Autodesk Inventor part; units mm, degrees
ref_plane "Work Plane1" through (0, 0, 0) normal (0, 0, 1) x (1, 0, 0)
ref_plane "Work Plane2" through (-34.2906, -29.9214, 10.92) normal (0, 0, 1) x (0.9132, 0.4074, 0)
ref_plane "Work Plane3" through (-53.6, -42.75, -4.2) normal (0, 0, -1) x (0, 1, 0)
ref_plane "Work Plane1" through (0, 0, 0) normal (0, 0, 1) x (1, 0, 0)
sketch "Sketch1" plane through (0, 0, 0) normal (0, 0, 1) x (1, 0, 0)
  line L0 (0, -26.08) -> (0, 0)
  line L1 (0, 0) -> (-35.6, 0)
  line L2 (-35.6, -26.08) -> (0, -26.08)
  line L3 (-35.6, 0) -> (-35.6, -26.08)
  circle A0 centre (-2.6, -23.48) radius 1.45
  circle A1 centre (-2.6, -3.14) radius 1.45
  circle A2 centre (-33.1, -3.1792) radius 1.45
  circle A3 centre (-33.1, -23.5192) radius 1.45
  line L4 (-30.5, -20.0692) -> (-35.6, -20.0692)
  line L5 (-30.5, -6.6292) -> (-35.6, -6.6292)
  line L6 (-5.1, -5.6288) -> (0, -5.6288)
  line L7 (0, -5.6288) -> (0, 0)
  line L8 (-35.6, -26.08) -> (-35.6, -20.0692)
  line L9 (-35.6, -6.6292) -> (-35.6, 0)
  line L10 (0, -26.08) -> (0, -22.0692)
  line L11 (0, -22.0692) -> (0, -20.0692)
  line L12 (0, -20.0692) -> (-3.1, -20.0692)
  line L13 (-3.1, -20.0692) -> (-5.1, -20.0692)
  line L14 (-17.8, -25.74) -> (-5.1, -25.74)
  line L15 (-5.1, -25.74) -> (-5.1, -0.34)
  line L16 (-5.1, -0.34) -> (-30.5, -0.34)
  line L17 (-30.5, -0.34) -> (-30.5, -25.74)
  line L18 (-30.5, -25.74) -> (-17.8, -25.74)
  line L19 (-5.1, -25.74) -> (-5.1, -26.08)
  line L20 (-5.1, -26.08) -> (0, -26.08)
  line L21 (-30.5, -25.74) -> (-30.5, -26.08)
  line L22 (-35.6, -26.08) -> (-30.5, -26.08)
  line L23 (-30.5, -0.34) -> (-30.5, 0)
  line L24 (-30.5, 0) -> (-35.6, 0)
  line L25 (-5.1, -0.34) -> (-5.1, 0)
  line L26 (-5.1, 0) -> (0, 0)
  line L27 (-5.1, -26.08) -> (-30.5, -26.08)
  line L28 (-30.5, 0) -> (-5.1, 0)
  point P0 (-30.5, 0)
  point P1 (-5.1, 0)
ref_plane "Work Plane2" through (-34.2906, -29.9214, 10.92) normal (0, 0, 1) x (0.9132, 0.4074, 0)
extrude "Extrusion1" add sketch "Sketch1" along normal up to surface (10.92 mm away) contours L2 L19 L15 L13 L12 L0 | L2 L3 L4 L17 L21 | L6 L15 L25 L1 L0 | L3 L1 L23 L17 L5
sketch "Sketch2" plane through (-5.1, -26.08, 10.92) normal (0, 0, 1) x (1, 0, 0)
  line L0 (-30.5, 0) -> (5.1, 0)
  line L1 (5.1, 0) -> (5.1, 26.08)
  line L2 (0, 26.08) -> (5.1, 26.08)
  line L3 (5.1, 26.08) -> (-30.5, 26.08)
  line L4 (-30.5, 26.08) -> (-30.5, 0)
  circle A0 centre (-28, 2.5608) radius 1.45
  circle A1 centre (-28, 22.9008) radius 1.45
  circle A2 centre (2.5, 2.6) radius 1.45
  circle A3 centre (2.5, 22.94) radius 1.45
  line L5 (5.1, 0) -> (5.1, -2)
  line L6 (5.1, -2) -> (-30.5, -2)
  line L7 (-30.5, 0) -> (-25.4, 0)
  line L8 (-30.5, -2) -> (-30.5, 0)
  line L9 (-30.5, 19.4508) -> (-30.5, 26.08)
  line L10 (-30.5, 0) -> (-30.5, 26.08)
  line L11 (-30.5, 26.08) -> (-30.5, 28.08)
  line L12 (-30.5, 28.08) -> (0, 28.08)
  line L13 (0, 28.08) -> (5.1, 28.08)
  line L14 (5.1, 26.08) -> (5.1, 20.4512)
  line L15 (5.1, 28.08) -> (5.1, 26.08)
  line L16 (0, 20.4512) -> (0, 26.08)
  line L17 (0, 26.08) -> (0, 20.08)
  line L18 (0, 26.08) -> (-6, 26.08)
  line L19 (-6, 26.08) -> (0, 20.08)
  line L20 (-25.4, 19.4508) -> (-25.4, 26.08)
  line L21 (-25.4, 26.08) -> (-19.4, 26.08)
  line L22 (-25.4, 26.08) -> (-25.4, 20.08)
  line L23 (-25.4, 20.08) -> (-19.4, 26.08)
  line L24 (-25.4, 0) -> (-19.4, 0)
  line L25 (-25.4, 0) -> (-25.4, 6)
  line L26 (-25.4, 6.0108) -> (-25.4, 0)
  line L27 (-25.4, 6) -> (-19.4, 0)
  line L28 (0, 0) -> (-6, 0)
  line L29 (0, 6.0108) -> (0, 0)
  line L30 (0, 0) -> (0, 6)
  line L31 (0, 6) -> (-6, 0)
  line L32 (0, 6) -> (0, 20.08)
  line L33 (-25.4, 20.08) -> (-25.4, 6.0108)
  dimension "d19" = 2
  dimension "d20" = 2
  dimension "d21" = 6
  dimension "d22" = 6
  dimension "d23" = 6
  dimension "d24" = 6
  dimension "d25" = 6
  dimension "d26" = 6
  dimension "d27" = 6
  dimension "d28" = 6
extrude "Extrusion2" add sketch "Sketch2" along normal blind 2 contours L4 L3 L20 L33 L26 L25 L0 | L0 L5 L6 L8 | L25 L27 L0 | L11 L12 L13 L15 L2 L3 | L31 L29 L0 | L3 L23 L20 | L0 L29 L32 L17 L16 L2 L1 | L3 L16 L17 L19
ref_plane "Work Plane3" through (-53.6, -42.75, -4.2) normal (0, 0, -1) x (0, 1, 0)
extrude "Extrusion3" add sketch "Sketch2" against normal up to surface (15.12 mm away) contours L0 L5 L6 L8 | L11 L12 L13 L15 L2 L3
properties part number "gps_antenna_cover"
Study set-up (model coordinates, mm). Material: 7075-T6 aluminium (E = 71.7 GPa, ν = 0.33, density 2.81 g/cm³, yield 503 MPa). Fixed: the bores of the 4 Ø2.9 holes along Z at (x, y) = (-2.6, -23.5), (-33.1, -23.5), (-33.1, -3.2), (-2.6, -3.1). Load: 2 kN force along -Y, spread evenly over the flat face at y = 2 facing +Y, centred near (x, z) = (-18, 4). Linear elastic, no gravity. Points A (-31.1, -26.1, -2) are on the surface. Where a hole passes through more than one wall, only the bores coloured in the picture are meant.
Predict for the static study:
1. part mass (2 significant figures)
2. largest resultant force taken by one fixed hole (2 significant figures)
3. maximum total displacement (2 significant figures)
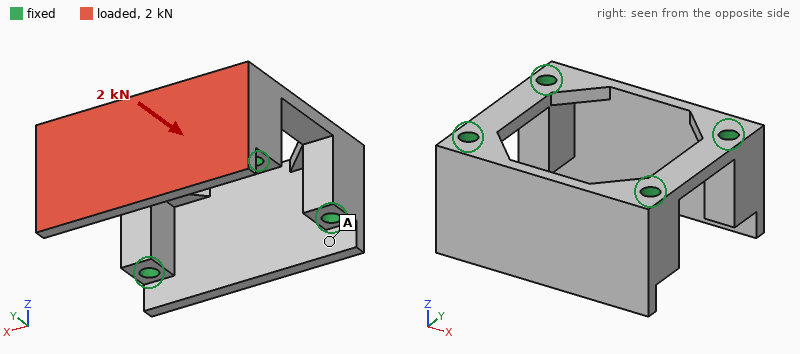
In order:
12 g
1.1 kN
0.15 mm
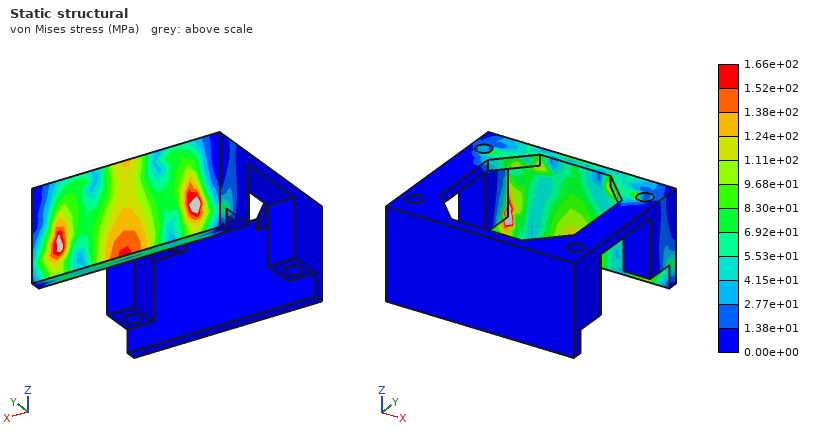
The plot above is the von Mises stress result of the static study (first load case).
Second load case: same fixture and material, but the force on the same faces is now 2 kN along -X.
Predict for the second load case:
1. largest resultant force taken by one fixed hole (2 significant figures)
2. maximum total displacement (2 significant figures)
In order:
1.0 kN
8.8 µm
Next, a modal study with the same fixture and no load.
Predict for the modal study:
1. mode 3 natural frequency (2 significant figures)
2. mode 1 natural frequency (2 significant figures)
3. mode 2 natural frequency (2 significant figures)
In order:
25 kHz
14 kHz
14 kHz
